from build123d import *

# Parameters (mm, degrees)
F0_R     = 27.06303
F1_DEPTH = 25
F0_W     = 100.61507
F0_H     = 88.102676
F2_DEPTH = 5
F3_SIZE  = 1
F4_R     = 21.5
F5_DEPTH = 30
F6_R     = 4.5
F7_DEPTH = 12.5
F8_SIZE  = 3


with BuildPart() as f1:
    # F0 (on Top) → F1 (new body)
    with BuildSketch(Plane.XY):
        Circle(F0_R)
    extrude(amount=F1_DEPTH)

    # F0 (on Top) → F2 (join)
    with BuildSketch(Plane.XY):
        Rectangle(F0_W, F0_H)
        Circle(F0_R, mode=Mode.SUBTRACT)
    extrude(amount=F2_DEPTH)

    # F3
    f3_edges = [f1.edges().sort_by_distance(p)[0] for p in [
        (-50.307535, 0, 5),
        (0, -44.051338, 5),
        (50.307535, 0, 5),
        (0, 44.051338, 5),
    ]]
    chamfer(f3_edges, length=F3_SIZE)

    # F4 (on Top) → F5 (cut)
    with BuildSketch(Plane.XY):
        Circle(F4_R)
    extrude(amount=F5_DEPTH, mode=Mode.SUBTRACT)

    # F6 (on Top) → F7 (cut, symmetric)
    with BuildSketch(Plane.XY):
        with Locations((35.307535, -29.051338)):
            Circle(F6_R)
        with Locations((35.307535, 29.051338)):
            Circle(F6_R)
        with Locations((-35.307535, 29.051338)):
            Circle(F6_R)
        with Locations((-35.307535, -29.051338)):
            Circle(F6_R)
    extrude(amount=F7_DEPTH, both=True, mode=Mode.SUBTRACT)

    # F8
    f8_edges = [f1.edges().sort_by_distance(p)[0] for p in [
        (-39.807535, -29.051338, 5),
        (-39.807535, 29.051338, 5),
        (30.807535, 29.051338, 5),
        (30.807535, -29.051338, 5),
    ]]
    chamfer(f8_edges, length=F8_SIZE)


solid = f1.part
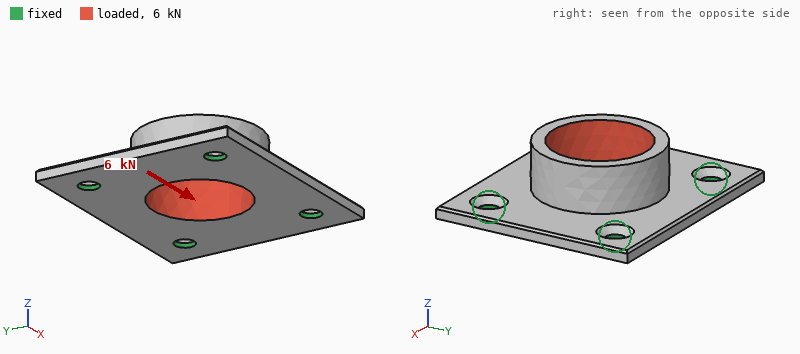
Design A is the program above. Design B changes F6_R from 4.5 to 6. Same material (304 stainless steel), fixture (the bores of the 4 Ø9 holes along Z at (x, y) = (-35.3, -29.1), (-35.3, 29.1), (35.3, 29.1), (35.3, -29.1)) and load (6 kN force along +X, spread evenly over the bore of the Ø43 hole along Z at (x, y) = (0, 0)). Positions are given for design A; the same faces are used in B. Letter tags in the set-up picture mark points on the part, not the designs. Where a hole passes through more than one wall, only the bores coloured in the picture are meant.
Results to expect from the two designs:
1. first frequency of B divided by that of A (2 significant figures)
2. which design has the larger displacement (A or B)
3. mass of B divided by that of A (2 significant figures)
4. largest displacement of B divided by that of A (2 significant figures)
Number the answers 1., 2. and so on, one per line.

1. 1.1
2. A
3. 0.98
4. 0.87
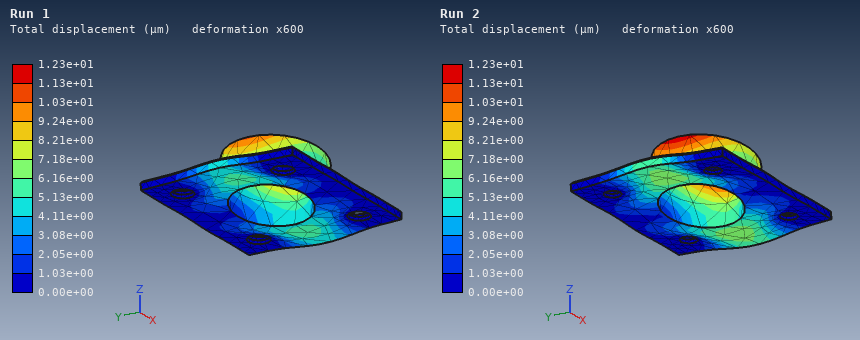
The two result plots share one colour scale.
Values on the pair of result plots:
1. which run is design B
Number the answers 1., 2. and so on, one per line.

1. Run 1
